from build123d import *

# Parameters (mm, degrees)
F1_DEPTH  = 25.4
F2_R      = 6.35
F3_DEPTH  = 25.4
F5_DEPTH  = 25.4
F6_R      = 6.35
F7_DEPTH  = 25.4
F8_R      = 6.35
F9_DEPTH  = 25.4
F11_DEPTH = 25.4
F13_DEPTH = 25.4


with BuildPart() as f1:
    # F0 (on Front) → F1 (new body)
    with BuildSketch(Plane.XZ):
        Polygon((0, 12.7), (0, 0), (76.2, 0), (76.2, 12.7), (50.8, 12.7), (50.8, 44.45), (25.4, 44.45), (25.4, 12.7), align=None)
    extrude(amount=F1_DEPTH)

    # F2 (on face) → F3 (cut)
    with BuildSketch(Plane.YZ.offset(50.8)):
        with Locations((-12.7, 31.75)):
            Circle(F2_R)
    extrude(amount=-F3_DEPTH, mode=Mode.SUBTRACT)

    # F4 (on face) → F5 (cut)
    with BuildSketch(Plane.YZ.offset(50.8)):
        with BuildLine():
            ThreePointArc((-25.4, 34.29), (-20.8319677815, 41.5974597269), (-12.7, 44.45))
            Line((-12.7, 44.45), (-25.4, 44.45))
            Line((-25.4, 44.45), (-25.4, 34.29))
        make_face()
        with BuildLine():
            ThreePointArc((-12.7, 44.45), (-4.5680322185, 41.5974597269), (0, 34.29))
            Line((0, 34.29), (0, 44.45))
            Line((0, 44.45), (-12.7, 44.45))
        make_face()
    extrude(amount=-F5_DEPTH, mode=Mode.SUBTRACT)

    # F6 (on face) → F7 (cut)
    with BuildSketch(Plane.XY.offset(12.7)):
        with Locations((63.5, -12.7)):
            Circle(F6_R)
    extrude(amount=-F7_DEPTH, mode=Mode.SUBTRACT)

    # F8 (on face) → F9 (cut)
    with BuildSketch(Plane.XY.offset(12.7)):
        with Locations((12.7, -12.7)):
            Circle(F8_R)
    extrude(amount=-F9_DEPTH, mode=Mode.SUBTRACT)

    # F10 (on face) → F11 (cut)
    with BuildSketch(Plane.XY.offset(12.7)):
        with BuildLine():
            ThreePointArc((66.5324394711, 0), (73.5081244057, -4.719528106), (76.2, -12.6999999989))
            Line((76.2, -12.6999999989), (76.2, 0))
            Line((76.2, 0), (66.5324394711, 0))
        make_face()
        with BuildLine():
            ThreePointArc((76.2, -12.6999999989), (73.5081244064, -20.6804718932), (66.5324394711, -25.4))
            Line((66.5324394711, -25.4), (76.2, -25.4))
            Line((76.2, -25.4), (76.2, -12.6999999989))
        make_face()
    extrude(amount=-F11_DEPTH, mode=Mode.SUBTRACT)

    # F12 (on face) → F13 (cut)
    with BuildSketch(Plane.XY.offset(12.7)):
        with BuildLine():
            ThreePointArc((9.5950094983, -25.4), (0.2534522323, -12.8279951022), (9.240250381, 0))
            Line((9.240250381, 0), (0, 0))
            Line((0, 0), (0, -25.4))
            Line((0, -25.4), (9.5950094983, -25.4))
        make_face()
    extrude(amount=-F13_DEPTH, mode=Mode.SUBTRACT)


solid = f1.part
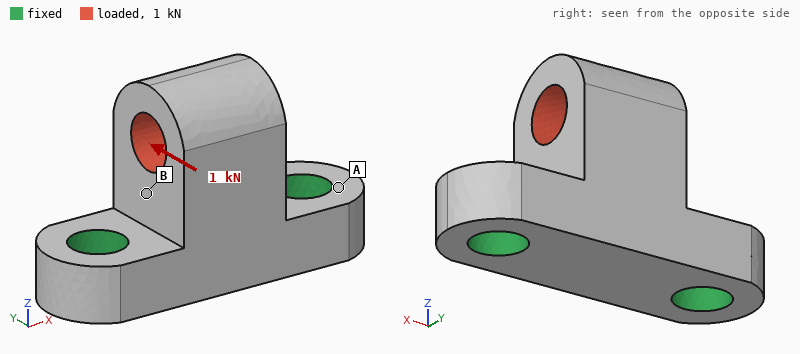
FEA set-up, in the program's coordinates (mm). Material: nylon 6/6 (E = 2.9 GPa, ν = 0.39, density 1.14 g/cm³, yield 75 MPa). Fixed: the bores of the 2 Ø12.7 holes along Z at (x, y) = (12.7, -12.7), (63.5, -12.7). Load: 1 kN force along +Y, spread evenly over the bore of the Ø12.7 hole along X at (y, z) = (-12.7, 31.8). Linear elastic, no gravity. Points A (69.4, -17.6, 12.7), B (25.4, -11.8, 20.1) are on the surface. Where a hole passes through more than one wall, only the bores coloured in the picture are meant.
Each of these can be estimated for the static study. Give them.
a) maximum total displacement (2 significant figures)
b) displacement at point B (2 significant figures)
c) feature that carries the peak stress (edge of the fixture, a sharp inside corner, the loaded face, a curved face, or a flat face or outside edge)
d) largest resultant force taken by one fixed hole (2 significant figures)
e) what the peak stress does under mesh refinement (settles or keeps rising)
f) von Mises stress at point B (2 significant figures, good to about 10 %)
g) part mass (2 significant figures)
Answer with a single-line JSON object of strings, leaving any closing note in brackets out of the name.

{"maximum total displacement": "0.53 mm", "displacement at point B": "0.18 mm", "feature that carries the peak stress": "edge of the fixture", "largest resultant force taken by one fixed hole": "500 N", "what the peak stress does under mesh refinement": "keeps rising", "von Mises stress at point B": "7.9 MPa", "part mass": "40 g"}
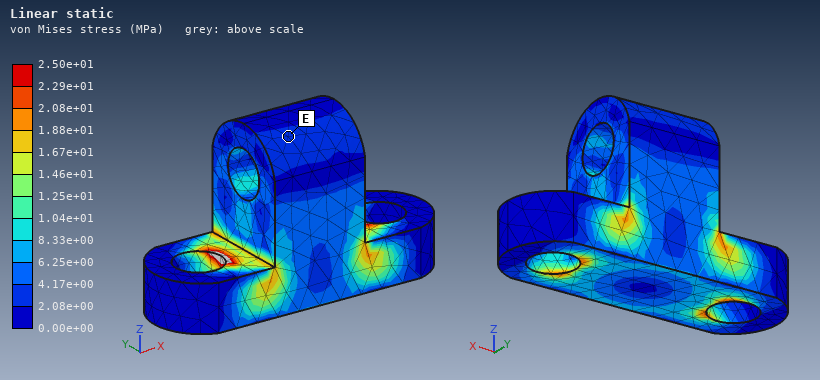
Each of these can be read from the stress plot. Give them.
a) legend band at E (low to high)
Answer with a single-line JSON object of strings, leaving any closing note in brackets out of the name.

{"legend band at E": "2.08e+00 to 4.17e+00 MPa"}
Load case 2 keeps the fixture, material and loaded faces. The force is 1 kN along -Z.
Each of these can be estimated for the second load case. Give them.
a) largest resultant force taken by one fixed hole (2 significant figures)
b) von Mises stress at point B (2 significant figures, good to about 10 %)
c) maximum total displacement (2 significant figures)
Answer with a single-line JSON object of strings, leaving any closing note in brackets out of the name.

{"largest resultant force taken by one fixed hole": "530 N", "von Mises stress at point B": "1.6 MPa", "maximum total displacement": "55 µm"}
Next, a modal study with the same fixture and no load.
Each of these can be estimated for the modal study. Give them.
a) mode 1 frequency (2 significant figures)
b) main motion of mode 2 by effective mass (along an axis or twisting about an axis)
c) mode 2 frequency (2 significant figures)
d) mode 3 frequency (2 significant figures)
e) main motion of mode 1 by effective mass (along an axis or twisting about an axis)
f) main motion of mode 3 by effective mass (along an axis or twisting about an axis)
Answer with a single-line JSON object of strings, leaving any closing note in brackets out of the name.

{"mode 1 frequency": "2200 Hz", "main motion of mode 2 by effective mass": "along X", "mode 2 frequency": "3800 Hz", "mode 3 frequency": "5300 Hz", "main motion of mode 1 by effective mass": "along Y", "main motion of mode 3 by effective mass": "along Z"}
